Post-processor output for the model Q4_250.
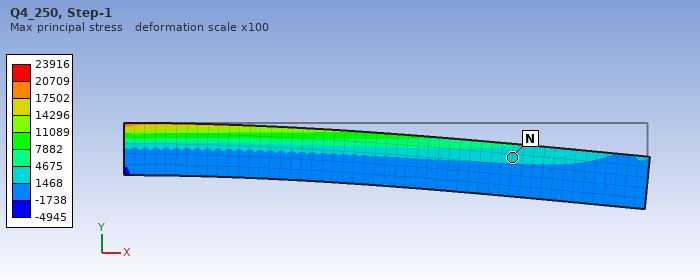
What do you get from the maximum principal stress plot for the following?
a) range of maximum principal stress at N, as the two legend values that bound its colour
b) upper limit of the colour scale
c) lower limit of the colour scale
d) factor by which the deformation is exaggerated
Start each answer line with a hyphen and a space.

- 1468 to 4675
- 23916
- -4945
- 100
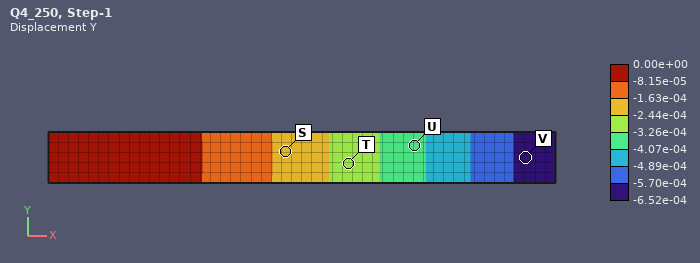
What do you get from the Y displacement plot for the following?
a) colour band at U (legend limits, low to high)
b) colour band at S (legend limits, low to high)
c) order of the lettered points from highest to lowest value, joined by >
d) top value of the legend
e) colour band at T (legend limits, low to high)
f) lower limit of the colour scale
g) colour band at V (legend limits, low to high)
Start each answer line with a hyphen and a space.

- -4.07e-04 to -3.26e-04
- -2.44e-04 to -1.63e-04
- S > T > U > V
- 0.00e+00
- -3.26e-04 to -2.44e-04
- -6.52e-04
- -6.52e-04 to -5.70e-04
